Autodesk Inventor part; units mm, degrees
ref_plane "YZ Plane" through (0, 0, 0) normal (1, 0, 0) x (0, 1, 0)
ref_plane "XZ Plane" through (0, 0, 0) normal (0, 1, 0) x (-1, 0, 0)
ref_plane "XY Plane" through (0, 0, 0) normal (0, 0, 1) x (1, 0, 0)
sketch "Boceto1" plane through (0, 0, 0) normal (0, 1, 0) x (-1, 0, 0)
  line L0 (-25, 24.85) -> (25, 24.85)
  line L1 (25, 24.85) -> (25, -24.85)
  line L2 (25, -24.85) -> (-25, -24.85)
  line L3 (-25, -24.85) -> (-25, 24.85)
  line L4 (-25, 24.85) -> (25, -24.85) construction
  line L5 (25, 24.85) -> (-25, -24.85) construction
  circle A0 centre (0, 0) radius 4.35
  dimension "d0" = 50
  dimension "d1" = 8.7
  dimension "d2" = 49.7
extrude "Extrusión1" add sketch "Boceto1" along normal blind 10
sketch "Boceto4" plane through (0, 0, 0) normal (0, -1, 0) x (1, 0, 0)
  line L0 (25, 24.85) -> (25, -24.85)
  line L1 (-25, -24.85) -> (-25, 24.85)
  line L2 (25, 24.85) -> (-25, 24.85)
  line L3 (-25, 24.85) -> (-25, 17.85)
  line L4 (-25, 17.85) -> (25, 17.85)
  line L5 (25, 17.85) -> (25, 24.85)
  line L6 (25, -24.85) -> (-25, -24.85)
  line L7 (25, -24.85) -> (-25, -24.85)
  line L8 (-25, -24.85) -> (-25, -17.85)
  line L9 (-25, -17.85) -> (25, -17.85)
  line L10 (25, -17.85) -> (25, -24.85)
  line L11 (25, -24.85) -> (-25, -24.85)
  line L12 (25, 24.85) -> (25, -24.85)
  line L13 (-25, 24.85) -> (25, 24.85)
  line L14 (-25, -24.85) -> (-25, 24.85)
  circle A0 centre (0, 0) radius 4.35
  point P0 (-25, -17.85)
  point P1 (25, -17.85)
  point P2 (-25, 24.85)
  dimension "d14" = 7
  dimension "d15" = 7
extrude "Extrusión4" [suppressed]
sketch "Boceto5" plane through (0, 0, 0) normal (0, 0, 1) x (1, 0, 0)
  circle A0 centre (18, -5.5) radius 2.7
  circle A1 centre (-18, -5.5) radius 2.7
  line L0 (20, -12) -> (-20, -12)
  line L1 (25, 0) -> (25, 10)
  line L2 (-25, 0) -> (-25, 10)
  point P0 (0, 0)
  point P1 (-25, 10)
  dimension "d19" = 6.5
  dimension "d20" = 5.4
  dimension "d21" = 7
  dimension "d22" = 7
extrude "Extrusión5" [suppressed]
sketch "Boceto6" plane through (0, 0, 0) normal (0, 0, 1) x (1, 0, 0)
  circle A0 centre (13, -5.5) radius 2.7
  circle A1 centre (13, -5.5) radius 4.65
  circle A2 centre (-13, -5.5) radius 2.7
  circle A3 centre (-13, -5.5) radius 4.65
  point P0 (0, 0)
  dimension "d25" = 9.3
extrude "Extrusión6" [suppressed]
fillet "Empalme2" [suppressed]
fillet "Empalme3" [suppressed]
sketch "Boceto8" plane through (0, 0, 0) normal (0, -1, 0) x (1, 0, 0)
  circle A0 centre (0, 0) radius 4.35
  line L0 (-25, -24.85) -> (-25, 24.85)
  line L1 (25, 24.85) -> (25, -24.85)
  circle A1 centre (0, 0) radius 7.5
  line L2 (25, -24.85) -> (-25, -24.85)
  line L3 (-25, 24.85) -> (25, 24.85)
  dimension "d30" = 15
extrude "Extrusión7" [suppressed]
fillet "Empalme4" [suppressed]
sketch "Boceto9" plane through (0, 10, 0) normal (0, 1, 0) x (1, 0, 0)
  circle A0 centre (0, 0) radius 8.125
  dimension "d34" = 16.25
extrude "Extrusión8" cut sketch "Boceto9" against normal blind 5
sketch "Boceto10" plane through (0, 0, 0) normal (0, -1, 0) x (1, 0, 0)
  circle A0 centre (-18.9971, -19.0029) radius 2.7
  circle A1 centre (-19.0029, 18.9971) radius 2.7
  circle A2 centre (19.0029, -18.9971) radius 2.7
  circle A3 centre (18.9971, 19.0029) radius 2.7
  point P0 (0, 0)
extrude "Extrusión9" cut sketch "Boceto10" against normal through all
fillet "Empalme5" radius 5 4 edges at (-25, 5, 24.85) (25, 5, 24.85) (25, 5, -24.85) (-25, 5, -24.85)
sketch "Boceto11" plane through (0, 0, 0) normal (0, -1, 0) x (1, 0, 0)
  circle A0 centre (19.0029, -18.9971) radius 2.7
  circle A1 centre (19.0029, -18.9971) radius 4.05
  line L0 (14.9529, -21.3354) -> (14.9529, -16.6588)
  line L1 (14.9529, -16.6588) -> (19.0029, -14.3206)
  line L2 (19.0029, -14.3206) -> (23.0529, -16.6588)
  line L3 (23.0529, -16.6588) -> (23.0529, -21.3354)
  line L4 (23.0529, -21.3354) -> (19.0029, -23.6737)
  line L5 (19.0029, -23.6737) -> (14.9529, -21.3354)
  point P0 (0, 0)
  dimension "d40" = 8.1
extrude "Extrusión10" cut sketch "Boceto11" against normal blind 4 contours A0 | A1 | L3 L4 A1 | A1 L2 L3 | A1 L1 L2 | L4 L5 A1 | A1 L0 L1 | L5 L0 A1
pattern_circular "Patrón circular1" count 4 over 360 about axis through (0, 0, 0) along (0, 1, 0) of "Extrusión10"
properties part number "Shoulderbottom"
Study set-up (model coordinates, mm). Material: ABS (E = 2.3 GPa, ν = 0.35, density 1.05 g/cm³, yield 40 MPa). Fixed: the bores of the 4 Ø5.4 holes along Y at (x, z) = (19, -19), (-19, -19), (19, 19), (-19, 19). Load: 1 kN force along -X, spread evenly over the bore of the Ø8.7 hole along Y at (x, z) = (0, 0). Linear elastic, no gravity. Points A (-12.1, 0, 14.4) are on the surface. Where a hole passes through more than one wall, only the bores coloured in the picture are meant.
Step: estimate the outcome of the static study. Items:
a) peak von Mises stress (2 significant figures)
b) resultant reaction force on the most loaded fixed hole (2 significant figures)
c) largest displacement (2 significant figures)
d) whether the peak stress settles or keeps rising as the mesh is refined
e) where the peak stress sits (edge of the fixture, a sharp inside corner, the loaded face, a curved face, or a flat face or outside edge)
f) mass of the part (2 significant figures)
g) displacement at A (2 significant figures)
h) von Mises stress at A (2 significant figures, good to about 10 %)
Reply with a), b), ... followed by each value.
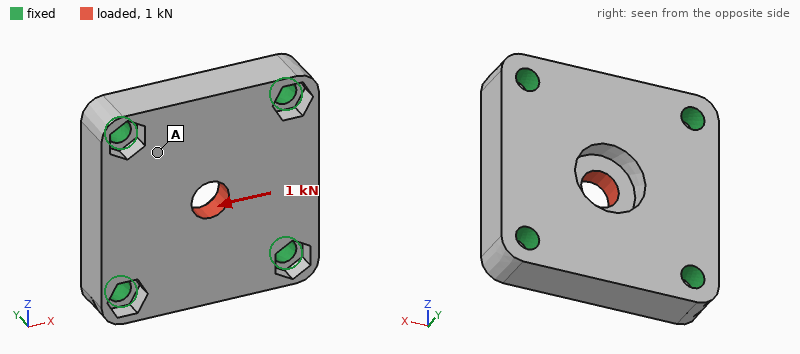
a) 13 MPa
b) 280 N
c) 52 µm
d) settles
e) the loaded face
f) 23 g
g) 14 µm
h) 1.7 MPa
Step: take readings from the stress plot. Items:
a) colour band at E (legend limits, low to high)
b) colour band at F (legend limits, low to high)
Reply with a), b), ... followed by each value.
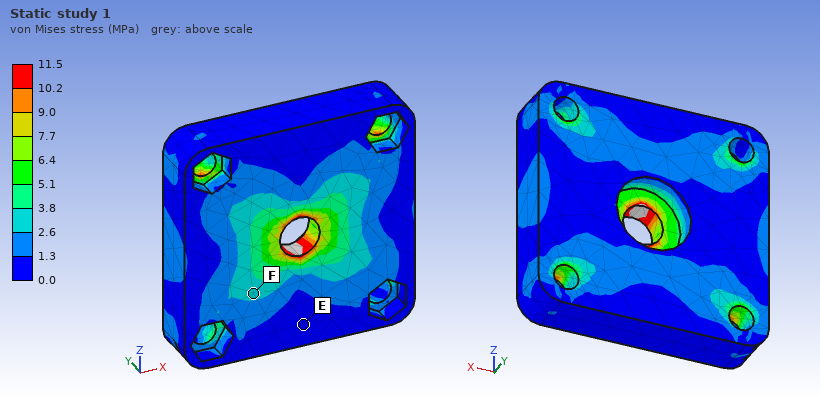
a) 0.0 to 1.3 MPa
b) 2.6 to 3.8 MPa
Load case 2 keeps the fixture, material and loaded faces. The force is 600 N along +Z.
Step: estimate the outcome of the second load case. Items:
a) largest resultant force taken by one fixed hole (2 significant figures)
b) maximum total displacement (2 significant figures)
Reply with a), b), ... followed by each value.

a) 170 N
b) 31 µm
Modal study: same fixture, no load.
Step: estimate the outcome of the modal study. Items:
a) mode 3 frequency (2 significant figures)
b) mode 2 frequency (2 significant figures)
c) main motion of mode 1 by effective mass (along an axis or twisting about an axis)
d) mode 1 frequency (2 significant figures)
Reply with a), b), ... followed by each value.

a) 7400 Hz
b) 7400 Hz
c) along Y
d) 5200 Hz
